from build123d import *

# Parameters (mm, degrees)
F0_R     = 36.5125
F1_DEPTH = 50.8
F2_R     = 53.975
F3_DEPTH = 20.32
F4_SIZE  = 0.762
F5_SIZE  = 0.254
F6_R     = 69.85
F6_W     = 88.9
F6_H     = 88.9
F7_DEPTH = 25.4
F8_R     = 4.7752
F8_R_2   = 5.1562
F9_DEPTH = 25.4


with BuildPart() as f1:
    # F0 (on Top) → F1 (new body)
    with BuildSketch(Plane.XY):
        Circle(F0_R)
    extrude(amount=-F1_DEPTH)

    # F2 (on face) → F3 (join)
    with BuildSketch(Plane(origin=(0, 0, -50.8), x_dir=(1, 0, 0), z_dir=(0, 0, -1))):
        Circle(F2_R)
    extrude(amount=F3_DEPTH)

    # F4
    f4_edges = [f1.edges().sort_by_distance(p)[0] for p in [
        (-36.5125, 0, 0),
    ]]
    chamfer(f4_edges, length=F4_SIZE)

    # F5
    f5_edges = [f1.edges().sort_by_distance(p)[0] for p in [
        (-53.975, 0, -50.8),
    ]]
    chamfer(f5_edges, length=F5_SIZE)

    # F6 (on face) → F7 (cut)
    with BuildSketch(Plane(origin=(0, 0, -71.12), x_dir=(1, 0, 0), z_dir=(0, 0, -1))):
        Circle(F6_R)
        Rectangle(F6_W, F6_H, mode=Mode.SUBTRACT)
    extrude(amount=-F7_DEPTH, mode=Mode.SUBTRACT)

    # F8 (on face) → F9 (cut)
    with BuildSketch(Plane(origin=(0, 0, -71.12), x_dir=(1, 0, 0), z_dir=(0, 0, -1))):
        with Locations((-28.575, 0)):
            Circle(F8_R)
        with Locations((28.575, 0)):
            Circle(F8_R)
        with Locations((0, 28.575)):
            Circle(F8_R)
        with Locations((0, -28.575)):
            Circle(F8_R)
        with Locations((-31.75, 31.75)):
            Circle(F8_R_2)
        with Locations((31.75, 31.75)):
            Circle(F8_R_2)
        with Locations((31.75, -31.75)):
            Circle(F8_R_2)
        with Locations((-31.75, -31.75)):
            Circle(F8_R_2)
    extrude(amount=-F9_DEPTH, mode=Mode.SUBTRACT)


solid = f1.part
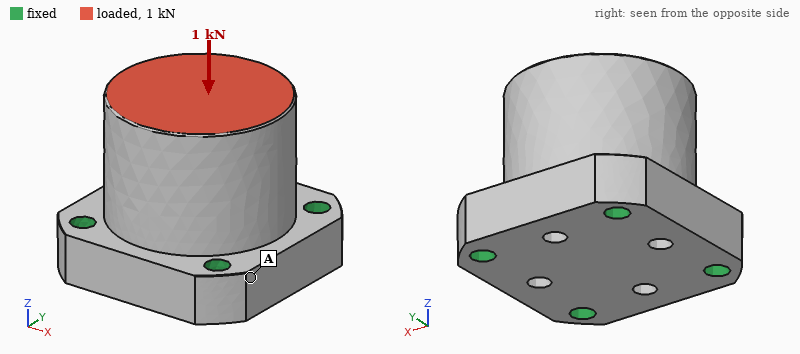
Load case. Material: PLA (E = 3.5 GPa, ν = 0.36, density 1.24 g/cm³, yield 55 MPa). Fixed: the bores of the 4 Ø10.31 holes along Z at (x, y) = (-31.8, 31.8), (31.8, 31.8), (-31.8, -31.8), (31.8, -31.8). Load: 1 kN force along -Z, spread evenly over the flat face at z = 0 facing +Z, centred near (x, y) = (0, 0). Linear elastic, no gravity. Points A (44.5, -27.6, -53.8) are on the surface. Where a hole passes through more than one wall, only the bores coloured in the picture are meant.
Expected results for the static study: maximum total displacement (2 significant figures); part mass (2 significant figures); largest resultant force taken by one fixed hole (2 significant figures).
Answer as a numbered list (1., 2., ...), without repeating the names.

1. 8.9 µm
2. 440 g
3. 260 N
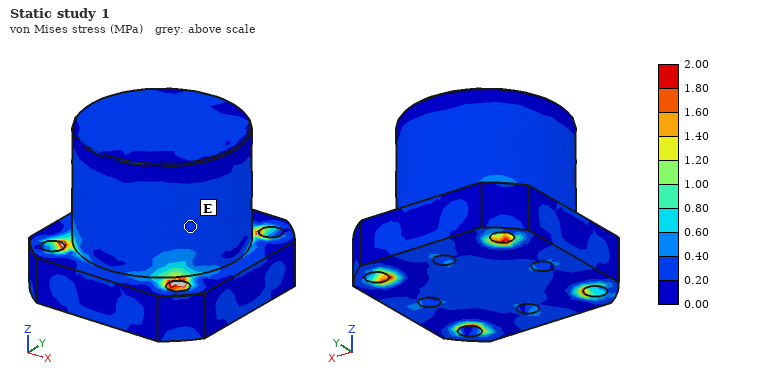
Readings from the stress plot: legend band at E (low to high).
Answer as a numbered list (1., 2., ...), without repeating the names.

1. 0.20 to 0.40 MPa
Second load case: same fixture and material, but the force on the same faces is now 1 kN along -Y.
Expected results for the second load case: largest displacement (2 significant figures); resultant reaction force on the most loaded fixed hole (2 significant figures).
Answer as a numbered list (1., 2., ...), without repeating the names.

1. 50 µm
2. 570 N
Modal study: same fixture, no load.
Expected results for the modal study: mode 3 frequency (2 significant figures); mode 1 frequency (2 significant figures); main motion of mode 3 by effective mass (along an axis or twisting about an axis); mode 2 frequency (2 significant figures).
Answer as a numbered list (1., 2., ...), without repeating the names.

1. 3300 Hz
2. 2200 Hz
3. along Z
4. 2200 Hz
